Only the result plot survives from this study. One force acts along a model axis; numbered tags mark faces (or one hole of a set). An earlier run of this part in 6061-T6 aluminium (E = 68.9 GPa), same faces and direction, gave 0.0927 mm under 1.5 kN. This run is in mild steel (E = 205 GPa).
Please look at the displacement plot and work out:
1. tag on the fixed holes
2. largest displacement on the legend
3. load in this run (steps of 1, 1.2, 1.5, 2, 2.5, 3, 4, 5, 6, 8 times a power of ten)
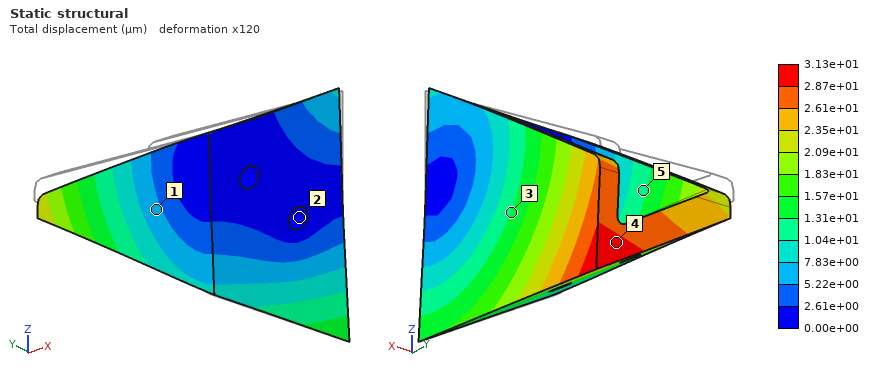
2
3.13e+01 µm
1.5 kN
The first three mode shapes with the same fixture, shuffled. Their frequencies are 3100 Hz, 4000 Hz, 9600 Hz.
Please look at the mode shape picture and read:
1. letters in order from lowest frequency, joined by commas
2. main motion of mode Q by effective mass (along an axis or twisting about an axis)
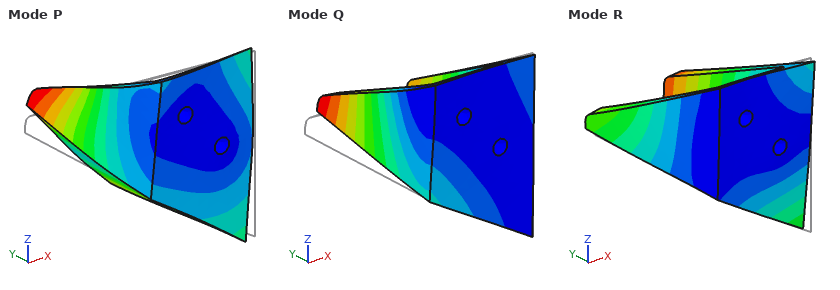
Q, R, P
along X
